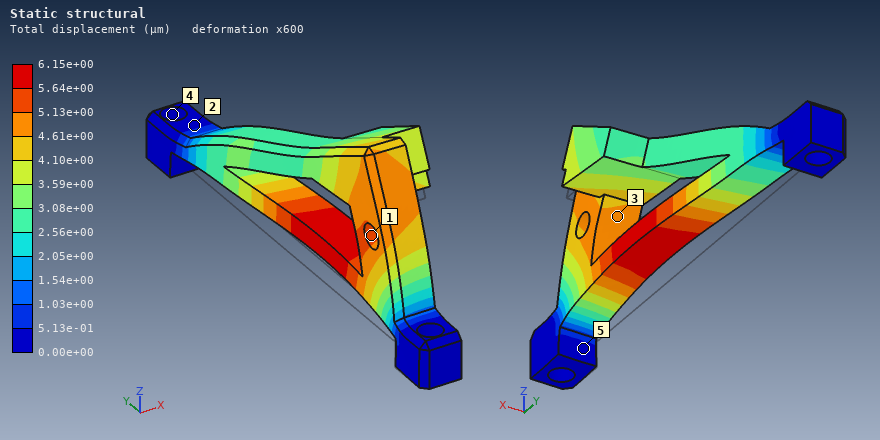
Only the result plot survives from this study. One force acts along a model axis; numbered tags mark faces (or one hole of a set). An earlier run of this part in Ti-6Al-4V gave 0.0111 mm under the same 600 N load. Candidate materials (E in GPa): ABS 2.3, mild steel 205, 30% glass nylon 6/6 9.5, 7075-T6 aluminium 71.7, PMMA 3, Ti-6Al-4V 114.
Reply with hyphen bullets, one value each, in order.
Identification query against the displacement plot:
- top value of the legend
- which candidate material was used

- 6.15e+00 µm
- mild steel
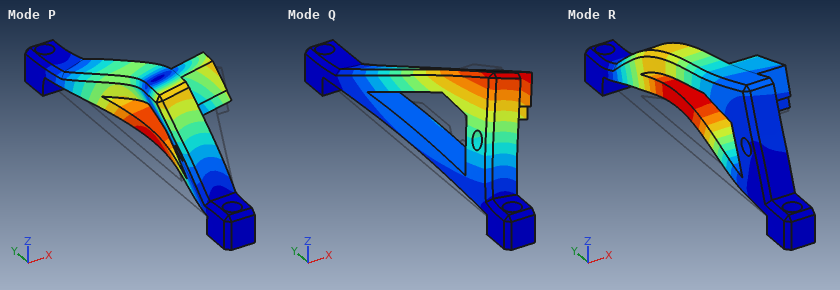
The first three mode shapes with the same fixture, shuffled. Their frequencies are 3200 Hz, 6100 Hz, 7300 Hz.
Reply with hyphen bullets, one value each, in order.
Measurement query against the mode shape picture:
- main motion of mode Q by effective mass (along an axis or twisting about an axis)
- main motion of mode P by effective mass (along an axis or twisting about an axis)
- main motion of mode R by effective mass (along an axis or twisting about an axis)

- along X
- along X
- along Z
